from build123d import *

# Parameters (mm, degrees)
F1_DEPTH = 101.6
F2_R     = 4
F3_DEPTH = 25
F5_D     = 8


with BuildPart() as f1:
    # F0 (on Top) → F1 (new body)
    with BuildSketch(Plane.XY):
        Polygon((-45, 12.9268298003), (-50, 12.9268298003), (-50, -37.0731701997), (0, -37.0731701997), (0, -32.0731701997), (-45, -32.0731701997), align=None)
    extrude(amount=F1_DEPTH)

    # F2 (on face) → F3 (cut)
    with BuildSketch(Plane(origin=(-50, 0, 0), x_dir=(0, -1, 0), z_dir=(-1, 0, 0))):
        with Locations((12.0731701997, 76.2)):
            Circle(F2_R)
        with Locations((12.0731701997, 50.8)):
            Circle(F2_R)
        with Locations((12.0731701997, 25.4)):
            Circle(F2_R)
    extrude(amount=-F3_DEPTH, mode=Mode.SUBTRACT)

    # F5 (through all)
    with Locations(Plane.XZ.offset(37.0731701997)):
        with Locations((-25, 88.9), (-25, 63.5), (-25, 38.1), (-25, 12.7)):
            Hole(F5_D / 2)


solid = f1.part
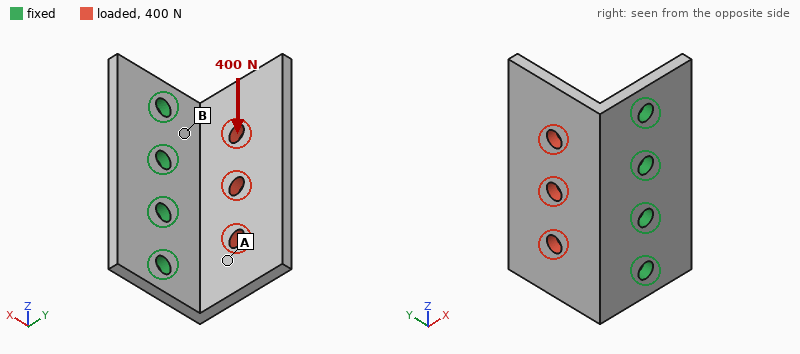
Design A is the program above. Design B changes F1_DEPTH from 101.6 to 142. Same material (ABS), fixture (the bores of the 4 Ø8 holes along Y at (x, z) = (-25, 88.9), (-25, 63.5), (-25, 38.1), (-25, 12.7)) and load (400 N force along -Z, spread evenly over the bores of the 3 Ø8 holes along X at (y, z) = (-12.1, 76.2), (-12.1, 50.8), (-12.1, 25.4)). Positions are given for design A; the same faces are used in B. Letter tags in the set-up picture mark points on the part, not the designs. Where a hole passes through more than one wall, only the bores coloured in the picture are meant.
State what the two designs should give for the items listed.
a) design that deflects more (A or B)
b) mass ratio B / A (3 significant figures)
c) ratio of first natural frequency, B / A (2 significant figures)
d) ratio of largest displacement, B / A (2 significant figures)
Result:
B
1.41
0.91
1.2
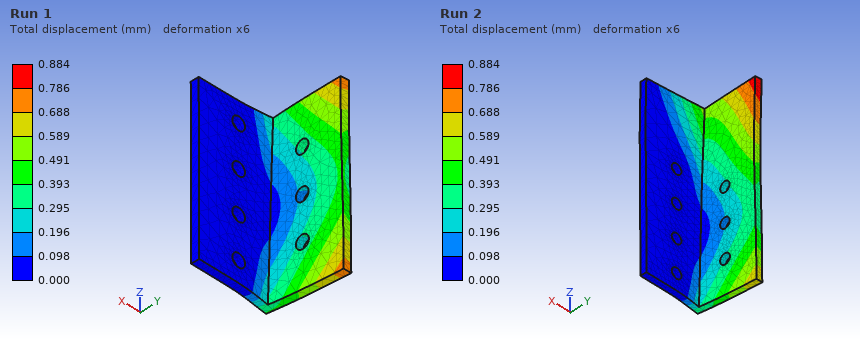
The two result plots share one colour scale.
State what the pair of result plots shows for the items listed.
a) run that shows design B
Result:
Run 2
